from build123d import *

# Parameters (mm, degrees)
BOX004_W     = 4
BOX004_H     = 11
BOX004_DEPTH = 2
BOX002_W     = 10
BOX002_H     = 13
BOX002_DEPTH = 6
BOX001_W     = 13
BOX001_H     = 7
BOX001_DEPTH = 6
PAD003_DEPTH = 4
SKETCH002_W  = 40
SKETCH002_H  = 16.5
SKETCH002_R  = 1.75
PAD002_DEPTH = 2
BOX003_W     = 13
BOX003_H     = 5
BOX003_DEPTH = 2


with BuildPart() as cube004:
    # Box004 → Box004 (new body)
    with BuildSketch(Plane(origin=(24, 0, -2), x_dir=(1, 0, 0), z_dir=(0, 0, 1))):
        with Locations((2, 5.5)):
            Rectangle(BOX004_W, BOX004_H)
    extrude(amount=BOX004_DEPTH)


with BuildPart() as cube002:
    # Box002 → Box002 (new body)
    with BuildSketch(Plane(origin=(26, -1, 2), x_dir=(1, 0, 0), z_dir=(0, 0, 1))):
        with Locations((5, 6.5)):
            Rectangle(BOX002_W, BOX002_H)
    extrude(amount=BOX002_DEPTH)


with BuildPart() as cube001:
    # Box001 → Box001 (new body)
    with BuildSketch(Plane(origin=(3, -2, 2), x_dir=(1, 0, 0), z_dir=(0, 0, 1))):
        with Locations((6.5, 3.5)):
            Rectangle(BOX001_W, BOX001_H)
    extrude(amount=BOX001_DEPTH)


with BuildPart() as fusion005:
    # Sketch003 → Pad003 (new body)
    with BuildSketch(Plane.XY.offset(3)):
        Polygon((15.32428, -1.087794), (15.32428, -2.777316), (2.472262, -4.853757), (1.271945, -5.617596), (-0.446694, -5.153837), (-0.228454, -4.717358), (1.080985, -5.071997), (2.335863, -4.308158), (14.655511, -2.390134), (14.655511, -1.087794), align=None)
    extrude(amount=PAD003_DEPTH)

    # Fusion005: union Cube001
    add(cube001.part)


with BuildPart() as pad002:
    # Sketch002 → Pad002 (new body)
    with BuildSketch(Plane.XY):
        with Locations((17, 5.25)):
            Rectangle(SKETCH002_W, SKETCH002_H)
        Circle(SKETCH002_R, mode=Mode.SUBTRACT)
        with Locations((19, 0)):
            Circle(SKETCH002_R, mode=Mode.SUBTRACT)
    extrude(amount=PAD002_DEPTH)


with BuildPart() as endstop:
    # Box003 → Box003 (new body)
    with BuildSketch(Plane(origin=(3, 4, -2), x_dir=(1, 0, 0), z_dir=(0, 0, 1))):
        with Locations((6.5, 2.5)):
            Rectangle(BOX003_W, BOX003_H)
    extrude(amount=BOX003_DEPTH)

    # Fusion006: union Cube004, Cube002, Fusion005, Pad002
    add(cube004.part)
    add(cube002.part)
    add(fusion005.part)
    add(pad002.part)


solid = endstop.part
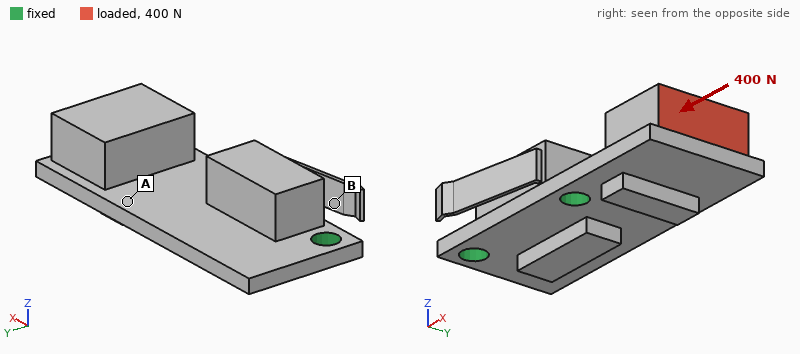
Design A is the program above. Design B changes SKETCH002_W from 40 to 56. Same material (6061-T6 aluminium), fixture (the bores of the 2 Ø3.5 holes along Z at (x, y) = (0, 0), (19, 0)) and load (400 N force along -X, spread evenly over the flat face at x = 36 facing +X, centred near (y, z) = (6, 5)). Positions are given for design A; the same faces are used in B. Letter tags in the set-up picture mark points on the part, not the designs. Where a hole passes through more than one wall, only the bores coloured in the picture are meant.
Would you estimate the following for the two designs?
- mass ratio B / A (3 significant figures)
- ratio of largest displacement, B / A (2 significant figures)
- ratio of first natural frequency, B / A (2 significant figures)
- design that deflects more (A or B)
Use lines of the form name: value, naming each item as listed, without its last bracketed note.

mass ratio B / A: 1.18
ratio of largest displacement, B / A: 1.5
ratio of first natural frequency, B / A: 1.0
design that deflects more: B
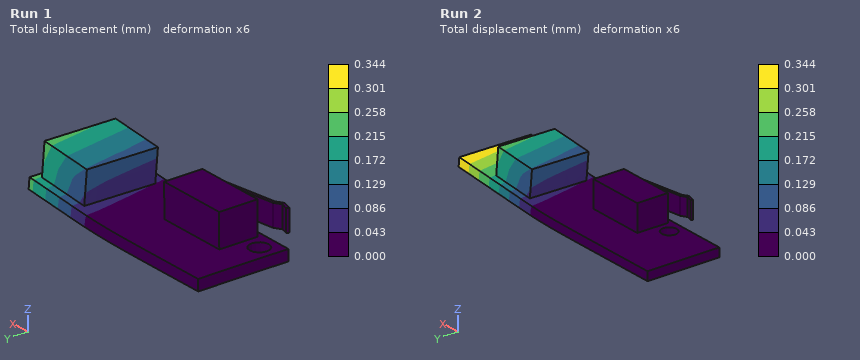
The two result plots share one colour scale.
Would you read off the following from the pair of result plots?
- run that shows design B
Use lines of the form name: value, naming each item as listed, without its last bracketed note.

run that shows design B: Run 2
